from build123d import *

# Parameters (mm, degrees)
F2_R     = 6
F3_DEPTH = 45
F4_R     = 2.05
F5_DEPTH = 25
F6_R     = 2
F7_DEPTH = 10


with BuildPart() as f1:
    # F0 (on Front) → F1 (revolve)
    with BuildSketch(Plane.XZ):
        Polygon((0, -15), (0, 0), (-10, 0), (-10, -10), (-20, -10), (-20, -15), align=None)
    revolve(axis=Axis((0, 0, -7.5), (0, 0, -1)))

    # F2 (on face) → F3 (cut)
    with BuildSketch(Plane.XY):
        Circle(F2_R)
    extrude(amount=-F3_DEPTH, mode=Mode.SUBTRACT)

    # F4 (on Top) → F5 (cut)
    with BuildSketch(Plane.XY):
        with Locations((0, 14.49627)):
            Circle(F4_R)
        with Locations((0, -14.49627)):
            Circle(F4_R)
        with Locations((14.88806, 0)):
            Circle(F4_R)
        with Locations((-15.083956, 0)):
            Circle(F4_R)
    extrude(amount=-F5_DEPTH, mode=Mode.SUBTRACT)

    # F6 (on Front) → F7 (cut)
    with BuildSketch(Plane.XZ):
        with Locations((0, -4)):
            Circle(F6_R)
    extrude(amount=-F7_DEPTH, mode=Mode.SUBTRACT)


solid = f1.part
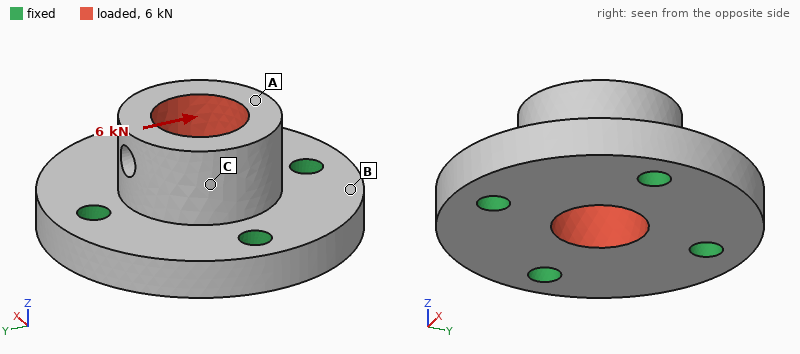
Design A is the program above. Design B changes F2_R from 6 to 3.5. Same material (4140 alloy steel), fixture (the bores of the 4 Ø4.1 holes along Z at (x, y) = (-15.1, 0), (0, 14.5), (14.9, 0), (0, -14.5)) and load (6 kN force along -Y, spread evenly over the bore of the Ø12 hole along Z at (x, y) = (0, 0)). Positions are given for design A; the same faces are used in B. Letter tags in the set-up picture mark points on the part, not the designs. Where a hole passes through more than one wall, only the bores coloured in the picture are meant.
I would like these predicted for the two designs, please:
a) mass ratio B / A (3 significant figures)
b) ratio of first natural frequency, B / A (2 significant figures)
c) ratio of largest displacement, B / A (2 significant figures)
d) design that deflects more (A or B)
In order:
1.15
0.95
0.80
A
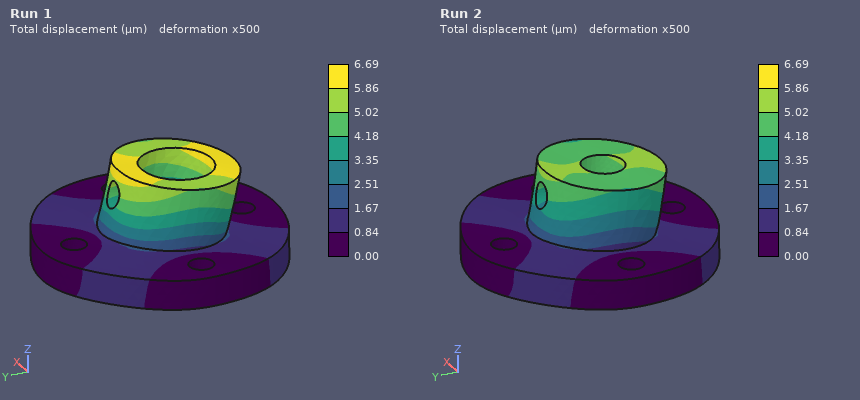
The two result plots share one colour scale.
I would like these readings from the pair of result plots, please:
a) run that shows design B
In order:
Run 2
